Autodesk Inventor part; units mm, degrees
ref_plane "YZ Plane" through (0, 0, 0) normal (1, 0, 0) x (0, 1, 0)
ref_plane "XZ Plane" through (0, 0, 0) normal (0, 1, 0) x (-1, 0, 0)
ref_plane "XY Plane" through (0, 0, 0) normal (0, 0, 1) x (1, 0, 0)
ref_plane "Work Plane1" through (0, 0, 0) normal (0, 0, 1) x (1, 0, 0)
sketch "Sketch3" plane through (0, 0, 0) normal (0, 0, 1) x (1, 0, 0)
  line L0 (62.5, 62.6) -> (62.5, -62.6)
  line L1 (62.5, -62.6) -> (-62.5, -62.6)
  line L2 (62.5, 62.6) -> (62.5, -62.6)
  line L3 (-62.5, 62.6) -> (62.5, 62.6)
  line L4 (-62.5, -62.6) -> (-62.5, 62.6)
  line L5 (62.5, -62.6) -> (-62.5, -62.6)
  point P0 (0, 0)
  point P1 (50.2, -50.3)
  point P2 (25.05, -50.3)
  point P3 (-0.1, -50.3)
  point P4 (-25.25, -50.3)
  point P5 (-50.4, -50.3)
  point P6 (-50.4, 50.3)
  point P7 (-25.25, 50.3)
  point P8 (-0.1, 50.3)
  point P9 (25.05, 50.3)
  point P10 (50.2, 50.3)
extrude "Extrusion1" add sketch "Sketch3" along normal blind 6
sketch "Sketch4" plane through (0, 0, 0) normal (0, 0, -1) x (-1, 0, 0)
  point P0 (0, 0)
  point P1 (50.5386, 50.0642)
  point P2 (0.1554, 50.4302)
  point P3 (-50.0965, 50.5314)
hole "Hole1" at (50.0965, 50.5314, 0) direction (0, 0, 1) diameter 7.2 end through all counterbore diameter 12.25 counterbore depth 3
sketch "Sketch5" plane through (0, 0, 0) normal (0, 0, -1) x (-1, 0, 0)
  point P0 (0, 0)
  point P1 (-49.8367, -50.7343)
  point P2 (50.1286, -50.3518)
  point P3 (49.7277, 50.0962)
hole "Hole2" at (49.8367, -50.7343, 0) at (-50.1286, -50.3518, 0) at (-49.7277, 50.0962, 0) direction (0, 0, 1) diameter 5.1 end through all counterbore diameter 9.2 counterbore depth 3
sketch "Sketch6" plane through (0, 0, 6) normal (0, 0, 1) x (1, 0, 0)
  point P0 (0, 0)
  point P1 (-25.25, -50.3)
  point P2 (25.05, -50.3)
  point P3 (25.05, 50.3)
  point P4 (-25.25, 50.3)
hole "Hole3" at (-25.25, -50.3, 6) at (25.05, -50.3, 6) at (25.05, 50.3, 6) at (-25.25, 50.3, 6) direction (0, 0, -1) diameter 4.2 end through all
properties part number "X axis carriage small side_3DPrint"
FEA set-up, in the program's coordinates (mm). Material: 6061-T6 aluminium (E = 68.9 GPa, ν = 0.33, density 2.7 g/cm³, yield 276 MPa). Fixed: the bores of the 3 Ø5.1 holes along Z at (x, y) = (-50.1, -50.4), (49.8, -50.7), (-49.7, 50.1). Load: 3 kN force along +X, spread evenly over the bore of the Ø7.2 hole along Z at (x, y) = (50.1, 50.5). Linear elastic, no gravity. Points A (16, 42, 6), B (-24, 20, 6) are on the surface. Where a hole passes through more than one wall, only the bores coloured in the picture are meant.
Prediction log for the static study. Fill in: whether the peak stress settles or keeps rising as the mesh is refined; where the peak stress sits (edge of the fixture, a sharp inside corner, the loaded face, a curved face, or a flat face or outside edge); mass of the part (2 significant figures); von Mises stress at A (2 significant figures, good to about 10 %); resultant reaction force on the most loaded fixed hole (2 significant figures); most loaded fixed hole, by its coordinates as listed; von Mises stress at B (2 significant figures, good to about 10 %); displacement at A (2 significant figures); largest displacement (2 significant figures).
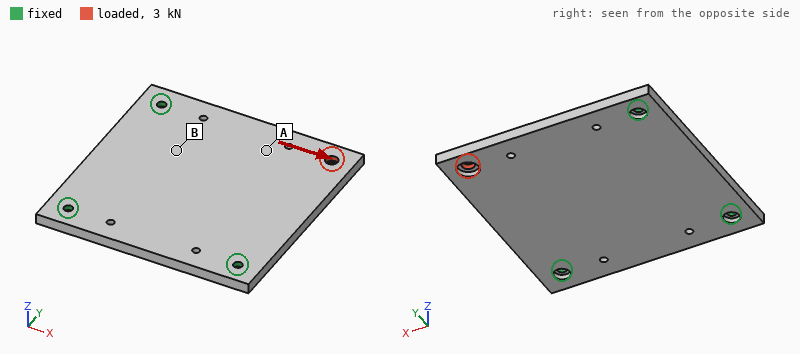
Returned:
keeps rising
edge of the fixture
250 g
19 MPa
2.2 kN
(-49.7, 50.1)
6.2 MPa
0.025 mm
0.15 mm
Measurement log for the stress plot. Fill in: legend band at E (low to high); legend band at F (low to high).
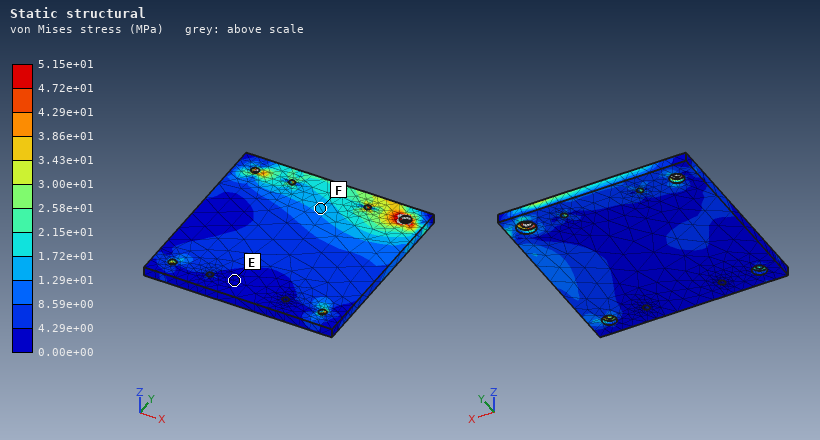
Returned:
0.00e+00 to 4.29e+00 MPa
1.29e+01 to 1.72e+01 MPa
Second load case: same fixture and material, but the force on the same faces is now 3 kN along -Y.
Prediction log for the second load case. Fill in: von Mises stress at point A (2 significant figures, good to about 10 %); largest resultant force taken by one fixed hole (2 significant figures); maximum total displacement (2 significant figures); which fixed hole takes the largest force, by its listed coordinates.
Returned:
11 MPa
2.1 kN
0.15 mm
(49.8, -50.7)
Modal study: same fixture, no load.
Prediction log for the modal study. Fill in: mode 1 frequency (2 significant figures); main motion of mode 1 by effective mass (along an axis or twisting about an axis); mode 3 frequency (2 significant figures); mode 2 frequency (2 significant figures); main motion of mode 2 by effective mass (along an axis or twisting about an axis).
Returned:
630 Hz
along Z
2300 Hz
1800 Hz
along Z
